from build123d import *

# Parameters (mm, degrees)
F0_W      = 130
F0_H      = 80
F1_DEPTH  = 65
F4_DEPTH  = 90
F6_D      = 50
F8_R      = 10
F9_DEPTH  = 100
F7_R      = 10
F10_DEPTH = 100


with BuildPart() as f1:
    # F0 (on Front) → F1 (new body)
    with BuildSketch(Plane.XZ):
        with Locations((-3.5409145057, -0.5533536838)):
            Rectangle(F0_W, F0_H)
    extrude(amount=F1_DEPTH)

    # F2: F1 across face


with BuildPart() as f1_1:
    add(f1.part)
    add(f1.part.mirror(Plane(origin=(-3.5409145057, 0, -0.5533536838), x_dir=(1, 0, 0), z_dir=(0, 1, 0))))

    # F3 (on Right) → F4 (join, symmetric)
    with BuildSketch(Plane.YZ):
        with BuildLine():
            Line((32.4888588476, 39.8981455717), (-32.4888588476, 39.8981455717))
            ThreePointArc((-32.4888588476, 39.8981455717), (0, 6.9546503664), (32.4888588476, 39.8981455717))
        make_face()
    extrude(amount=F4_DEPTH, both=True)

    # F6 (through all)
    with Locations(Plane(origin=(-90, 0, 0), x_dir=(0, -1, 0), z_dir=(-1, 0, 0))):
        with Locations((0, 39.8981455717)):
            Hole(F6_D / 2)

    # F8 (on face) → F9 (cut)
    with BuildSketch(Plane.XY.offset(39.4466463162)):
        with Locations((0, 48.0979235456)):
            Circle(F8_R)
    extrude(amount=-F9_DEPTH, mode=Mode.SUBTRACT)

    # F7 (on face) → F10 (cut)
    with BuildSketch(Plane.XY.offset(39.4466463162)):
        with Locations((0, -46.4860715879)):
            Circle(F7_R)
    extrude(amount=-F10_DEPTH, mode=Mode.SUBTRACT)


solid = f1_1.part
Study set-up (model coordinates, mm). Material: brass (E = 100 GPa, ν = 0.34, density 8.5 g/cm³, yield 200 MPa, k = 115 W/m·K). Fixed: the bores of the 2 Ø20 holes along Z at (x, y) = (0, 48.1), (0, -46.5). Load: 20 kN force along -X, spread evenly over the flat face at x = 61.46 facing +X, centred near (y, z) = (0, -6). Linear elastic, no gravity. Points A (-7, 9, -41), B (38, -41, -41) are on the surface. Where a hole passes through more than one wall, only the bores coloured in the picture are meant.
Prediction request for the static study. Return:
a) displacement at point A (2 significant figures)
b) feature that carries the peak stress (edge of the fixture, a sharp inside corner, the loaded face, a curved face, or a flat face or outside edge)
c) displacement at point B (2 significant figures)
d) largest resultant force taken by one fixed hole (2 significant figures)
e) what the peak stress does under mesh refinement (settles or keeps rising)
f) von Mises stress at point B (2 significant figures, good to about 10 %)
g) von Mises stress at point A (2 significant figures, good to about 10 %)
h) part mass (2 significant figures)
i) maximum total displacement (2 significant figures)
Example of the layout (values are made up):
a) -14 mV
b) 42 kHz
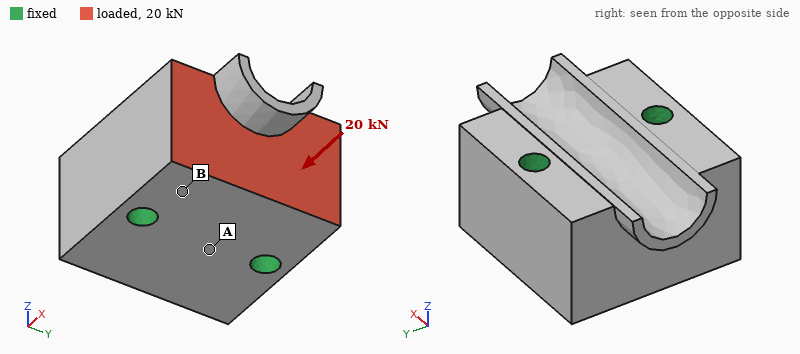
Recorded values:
a) 0.74 µm
b) edge of the fixture
c) 1.1 µm
d) 10 kN
e) keeps rising
f) 2.7 MPa
g) 1.00 MPa
h) 10 kg
i) 2.0 µm
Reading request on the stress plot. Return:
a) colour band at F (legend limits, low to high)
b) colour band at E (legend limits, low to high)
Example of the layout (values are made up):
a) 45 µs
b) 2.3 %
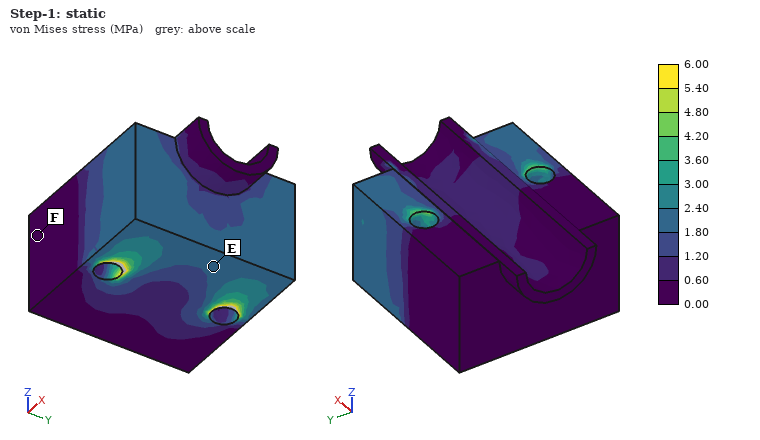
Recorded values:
a) 0.00 to 0.60 MPa
b) 1.80 to 2.40 MPa
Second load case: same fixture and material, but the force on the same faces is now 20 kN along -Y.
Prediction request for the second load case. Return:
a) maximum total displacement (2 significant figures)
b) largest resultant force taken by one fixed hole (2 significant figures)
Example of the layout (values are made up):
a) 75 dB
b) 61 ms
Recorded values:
a) 7.5 µm
b) 15 kN
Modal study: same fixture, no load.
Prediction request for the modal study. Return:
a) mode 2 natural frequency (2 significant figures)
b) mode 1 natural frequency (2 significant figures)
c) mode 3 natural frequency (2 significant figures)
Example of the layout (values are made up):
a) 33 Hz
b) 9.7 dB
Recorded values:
a) 5500 Hz
b) 5100 Hz
c) 5700 Hz
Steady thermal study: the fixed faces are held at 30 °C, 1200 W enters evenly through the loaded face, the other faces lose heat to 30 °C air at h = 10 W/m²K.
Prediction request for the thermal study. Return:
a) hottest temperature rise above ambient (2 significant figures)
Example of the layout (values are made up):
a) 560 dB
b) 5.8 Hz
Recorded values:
a) 71 K
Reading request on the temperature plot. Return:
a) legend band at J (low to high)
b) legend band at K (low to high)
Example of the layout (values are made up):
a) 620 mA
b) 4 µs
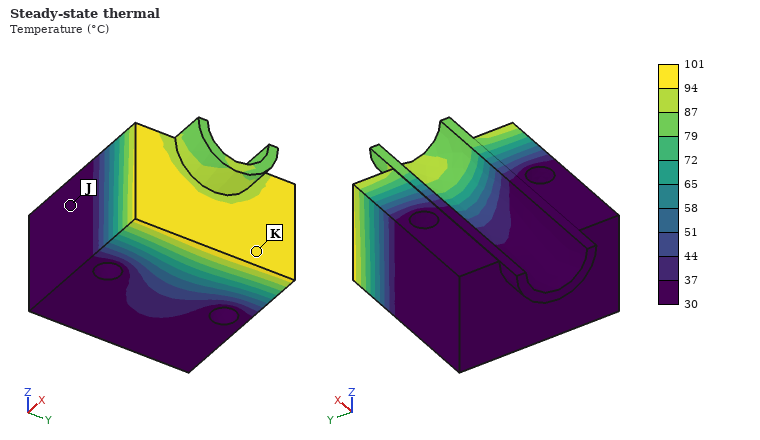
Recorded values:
a) 30 to 37 °C
b) 94 to 101 °C
